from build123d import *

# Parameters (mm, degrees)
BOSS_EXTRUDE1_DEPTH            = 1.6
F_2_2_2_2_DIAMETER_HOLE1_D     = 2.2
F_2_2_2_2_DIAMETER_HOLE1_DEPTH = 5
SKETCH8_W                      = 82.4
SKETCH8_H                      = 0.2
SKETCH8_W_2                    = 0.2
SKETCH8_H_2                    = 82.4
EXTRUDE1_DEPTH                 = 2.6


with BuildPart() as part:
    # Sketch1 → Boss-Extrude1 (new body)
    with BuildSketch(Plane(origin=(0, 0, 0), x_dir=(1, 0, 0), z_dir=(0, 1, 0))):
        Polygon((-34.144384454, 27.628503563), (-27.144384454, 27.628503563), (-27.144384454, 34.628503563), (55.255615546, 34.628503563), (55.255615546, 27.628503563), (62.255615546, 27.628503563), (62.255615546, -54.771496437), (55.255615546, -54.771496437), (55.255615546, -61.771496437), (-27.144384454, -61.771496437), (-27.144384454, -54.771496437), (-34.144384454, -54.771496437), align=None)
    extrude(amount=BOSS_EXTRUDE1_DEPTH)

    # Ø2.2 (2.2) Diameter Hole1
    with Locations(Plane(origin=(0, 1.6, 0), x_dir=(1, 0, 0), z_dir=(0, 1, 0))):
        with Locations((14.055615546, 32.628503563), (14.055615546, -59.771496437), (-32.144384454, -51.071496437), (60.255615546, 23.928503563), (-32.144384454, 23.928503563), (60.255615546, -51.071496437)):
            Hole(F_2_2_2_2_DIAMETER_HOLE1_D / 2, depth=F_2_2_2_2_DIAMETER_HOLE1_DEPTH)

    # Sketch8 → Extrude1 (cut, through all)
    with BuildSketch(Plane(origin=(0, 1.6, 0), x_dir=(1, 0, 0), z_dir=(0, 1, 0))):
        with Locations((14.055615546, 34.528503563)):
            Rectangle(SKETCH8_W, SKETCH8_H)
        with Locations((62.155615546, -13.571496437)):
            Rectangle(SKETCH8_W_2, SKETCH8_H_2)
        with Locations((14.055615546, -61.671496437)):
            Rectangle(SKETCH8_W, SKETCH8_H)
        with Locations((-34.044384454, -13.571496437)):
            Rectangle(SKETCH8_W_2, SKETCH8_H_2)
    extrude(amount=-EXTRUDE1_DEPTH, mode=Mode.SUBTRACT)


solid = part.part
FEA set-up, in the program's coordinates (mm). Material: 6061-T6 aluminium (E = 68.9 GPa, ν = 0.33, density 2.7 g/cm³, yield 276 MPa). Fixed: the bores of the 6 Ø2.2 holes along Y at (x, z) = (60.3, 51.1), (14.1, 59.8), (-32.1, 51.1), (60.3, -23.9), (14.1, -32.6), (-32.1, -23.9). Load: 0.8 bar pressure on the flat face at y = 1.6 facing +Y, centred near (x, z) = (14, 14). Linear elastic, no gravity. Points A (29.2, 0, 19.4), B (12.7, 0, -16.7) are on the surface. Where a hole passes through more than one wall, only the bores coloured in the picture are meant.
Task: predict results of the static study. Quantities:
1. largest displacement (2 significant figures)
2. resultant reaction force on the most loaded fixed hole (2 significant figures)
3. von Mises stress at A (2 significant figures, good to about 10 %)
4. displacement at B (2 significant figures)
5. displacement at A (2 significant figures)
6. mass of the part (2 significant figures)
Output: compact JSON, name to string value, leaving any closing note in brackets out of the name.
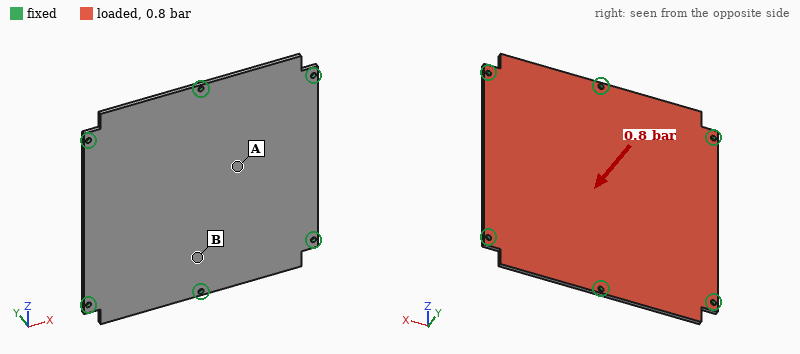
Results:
{"largest displacement": "0.75 mm", "resultant reaction force on the most loaded fixed hole": "160 N", "von Mises stress at A": "61 MPa", "displacement at B": "0.31 mm", "displacement at A": "0.70 mm", "mass of the part": "39 g"}
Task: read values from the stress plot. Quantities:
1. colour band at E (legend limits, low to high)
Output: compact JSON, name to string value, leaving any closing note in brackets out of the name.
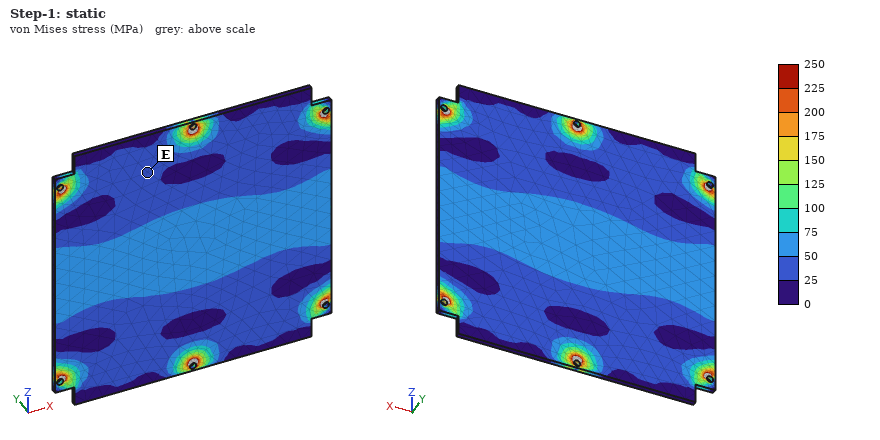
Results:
{"colour band at E": "25 to 50 MPa"}
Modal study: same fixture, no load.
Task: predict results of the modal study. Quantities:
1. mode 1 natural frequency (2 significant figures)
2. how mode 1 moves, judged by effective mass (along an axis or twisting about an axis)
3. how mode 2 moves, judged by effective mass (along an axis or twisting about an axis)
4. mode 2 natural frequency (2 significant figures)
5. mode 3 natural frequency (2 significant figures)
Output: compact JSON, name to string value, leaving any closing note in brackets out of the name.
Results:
{"mode 1 natural frequency": "940 Hz", "how mode 1 moves, judged by effective mass": "along Y", "how mode 2 moves, judged by effective mass": "twisting about Z", "mode 2 natural frequency": "1400 Hz", "mode 3 natural frequency": "2100 Hz"}
